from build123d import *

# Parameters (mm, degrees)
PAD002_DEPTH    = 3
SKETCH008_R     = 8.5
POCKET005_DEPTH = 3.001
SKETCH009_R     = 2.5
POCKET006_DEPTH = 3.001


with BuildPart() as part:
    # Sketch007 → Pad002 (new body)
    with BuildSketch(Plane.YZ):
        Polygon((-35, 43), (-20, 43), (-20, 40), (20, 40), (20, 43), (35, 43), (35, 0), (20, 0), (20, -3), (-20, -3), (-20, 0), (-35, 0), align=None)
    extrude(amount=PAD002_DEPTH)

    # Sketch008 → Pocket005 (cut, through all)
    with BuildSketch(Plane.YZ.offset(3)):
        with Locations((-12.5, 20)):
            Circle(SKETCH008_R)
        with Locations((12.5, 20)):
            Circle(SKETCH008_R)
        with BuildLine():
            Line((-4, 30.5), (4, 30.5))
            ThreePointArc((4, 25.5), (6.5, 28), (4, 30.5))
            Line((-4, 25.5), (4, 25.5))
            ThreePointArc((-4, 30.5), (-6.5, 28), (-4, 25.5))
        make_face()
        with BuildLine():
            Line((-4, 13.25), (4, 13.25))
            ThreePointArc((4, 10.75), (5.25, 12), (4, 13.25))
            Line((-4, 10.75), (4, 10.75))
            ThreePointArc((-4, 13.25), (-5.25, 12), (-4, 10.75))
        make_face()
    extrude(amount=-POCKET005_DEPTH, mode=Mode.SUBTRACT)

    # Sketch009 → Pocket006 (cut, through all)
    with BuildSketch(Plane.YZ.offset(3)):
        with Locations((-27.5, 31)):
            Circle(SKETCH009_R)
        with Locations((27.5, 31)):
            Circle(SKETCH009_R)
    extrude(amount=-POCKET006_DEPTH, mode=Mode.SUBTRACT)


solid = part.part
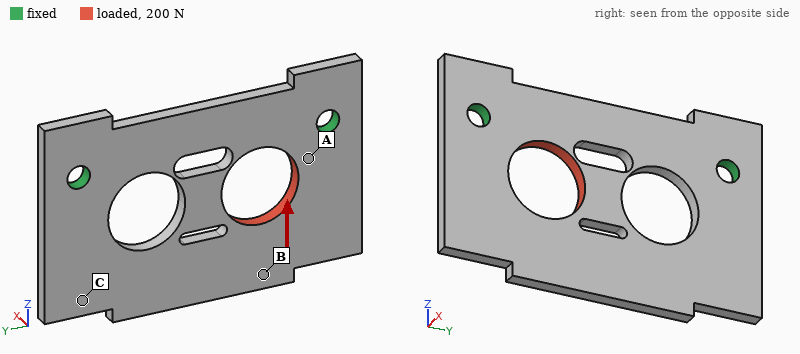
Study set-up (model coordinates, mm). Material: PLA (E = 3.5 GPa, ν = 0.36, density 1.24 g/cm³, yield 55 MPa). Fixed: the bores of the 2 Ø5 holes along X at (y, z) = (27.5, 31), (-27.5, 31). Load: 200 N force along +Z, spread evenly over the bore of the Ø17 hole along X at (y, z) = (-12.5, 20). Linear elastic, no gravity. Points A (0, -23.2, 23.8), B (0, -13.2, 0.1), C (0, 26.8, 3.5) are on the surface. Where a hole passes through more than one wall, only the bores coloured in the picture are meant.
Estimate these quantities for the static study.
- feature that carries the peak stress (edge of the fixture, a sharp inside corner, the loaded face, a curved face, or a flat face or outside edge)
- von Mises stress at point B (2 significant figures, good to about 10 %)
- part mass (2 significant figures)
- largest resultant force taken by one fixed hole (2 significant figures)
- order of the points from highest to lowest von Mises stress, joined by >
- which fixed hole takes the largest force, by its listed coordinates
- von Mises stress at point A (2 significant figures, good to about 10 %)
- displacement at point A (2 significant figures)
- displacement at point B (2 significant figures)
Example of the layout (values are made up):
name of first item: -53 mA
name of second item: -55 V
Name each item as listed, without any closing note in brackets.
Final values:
feature that carries the peak stress: a curved face
von Mises stress at point B: 2.1 MPa
part mass: 9.0 g
largest resultant force taken by one fixed hole: 150 N
order of the points from highest to lowest von Mises stress, joined by >: A > B > C
which fixed hole takes the largest force, by its listed coordinates: (-27.5, 31)
von Mises stress at point A: 4.4 MPa
displacement at point A: 10 µm
displacement at point B: 31 µm
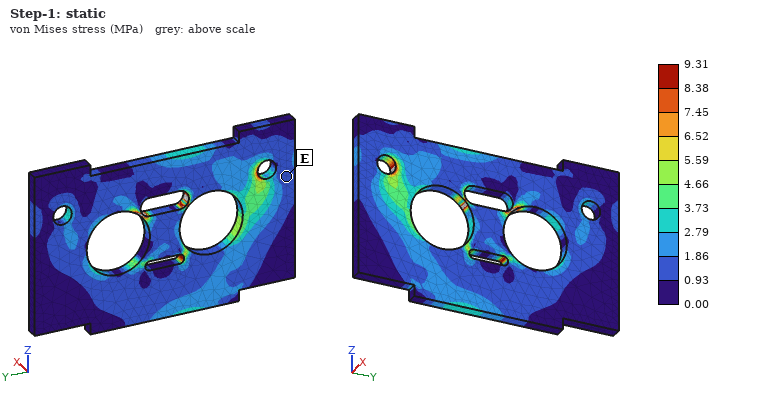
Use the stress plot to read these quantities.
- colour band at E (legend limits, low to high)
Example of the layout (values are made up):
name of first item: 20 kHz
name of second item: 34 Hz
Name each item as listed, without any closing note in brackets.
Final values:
colour band at E: 0.93 to 1.86 MPa
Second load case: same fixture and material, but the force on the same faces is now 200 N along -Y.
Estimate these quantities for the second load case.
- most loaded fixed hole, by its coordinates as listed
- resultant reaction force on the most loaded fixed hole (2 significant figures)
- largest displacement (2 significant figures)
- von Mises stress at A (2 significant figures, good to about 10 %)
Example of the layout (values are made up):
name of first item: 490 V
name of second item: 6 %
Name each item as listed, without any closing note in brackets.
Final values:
most loaded fixed hole, by its coordinates as listed: (-27.5, 31)
resultant reaction force on the most loaded fixed hole: 140 N
largest displacement: 51 µm
von Mises stress at A: 2.7 MPa
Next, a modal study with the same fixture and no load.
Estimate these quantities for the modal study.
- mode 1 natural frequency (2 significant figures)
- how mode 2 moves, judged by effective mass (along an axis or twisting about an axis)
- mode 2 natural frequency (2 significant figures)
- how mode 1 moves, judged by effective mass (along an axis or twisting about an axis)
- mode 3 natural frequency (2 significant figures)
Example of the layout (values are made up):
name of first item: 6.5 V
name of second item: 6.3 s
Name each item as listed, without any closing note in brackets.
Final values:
mode 1 natural frequency: 540 Hz
how mode 2 moves, judged by effective mass: twisting about Z
mode 2 natural frequency: 1100 Hz
how mode 1 moves, judged by effective mass: along X
mode 3 natural frequency: 1700 Hz
